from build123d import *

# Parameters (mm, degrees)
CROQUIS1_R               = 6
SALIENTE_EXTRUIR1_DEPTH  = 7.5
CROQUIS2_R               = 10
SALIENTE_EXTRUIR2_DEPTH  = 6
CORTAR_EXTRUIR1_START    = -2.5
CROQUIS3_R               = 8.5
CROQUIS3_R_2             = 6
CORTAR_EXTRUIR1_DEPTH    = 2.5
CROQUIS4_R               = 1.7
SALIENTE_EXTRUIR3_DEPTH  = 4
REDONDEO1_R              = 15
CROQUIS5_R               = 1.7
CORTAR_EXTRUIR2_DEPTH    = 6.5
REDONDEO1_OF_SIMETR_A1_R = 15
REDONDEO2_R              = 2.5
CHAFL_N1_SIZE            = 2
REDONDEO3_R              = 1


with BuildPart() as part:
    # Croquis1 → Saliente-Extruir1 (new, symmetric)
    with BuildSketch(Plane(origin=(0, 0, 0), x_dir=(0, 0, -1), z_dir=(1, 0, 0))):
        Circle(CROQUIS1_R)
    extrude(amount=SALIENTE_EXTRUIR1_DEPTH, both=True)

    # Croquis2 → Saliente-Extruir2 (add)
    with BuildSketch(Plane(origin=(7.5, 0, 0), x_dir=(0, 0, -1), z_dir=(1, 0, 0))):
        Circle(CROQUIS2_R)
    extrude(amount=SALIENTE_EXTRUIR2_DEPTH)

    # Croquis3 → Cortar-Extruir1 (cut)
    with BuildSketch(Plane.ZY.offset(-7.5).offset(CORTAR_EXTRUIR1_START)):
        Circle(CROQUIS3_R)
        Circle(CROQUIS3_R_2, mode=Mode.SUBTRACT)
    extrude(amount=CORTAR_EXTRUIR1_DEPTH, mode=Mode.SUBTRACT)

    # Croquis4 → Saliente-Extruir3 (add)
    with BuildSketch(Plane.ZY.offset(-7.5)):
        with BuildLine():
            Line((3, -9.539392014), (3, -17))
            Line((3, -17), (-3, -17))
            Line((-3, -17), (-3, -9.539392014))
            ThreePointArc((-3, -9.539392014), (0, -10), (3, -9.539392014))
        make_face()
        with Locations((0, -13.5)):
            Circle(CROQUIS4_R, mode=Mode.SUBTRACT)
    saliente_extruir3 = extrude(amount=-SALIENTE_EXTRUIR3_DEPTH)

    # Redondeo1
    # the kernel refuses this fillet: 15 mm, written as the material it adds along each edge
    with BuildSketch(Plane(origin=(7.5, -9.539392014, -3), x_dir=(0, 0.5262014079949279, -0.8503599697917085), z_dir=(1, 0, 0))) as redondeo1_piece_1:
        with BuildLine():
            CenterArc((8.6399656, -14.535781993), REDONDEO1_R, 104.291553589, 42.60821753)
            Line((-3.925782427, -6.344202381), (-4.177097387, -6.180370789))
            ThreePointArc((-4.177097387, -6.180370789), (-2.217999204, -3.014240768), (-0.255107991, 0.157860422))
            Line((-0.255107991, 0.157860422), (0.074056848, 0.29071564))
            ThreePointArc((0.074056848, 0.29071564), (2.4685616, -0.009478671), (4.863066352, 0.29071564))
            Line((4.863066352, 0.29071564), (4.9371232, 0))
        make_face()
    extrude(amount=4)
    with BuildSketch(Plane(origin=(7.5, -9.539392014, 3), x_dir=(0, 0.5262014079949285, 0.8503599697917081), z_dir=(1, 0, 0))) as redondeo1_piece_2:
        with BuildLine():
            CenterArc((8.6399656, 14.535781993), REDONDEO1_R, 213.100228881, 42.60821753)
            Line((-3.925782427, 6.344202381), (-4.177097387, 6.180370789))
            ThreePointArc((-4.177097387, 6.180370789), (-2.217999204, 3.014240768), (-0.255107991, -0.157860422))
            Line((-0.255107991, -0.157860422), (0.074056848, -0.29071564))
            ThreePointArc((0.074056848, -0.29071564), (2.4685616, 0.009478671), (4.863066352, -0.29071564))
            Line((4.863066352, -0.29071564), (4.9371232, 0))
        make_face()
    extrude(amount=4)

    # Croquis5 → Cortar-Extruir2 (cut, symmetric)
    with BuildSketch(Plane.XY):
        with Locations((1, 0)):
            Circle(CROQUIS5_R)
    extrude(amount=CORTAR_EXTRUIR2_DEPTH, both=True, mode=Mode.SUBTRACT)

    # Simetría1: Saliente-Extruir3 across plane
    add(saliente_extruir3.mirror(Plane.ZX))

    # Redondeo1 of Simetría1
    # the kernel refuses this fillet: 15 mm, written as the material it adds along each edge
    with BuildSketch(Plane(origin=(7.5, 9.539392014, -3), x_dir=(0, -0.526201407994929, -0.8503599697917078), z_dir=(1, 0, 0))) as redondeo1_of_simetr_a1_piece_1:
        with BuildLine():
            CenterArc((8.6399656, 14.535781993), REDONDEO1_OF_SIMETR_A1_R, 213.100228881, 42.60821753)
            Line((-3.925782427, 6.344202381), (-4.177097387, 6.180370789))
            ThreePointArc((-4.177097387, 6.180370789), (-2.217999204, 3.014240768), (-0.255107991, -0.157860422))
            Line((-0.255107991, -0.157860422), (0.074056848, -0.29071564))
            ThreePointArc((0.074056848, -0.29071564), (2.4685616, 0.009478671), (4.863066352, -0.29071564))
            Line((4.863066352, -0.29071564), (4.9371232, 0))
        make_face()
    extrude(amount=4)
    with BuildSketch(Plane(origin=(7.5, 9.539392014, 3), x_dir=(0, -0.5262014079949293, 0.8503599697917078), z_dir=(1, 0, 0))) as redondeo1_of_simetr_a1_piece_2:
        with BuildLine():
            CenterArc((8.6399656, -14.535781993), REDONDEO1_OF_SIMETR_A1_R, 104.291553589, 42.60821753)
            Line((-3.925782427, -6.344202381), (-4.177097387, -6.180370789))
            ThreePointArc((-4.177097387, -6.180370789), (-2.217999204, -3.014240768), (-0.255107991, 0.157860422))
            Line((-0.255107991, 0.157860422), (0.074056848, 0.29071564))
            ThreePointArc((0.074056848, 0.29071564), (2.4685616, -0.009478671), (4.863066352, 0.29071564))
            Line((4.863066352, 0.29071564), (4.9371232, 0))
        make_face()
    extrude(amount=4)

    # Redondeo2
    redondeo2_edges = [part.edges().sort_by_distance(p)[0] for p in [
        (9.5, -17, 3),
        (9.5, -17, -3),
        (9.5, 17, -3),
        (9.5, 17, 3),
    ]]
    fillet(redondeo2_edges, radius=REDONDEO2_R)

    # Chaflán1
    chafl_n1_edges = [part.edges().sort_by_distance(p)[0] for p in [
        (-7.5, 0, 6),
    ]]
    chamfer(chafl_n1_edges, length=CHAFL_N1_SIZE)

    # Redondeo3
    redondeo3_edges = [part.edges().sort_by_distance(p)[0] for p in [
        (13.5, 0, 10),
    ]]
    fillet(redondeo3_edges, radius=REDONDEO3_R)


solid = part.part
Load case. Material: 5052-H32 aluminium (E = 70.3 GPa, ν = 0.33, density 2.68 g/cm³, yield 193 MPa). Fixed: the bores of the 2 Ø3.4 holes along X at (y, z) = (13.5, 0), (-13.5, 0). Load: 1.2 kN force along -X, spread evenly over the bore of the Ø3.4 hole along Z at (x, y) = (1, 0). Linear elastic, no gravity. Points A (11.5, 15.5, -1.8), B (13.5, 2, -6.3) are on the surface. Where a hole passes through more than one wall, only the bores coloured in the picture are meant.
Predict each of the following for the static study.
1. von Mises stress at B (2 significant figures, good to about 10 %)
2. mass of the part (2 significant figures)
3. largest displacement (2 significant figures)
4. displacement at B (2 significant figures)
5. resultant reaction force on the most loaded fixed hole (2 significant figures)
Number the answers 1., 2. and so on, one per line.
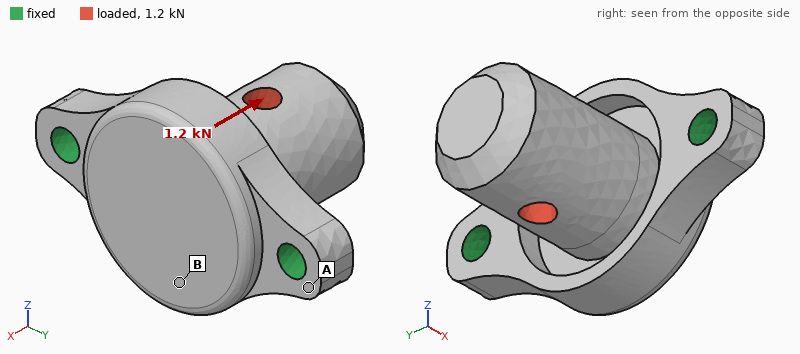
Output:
1. 33 MPa
2. 9.3 g
3. 16 µm
4. 14 µm
5. 770 N
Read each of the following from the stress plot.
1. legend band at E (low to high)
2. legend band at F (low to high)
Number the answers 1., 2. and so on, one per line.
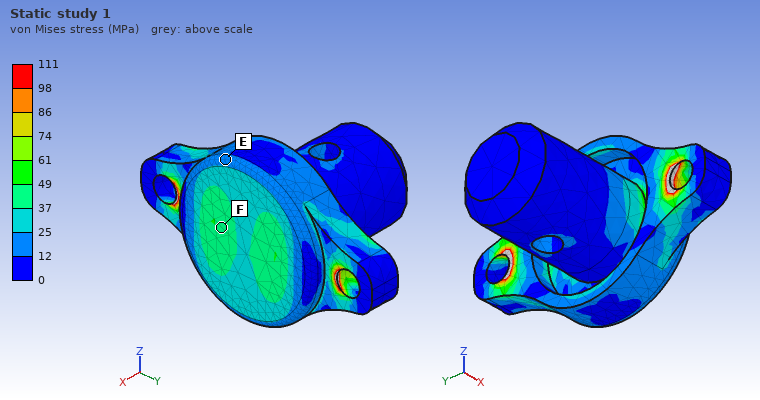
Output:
1. 12 to 25 MPa
2. 37 to 49 MPa
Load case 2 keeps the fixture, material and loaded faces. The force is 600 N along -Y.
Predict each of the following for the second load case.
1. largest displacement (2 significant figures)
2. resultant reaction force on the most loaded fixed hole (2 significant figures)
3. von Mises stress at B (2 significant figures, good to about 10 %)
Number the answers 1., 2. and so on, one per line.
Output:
1. 29 µm
2. 420 N
3. 10 MPa
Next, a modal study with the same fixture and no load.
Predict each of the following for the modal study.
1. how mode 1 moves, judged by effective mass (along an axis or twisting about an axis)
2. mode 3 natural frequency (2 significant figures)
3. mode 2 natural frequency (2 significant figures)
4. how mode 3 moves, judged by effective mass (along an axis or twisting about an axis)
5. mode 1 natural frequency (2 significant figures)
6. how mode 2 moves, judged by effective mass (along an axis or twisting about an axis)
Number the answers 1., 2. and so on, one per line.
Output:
1. along Z
2. 17 kHz
3. 12 kHz
4. along X
5. 7100 Hz
6. along Y
